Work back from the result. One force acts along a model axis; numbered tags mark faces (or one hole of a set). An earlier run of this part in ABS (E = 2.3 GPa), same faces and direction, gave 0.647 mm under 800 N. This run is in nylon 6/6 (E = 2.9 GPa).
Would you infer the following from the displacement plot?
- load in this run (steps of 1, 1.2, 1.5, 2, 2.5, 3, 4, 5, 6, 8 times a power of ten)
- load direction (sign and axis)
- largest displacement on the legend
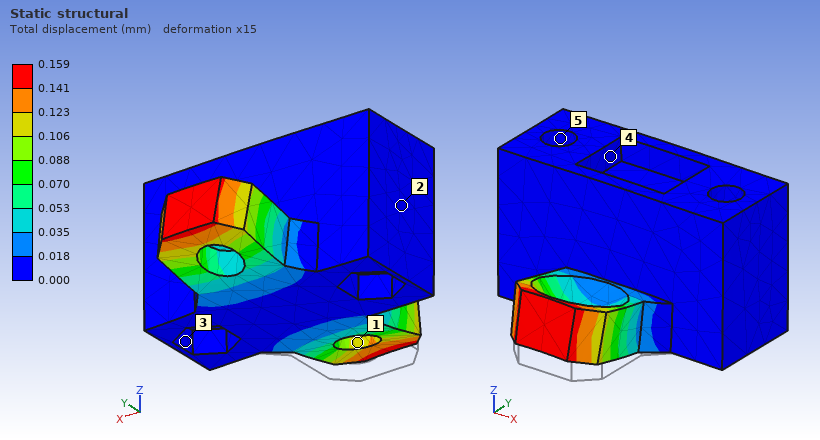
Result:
250 N
+Z
0.159 mm
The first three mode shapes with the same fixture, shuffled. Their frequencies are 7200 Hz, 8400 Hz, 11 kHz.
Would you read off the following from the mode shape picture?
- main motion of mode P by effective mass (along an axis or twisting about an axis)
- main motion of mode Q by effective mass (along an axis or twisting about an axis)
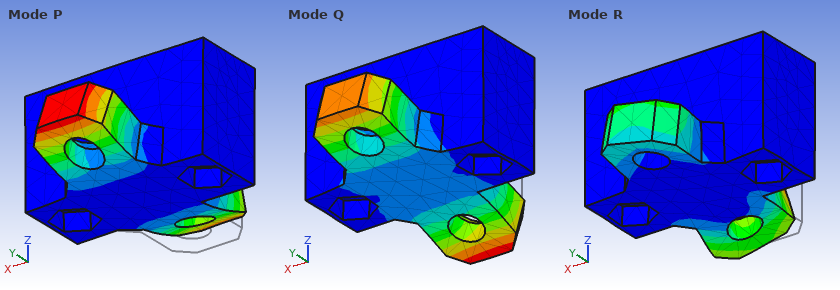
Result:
along Z
twisting about X
